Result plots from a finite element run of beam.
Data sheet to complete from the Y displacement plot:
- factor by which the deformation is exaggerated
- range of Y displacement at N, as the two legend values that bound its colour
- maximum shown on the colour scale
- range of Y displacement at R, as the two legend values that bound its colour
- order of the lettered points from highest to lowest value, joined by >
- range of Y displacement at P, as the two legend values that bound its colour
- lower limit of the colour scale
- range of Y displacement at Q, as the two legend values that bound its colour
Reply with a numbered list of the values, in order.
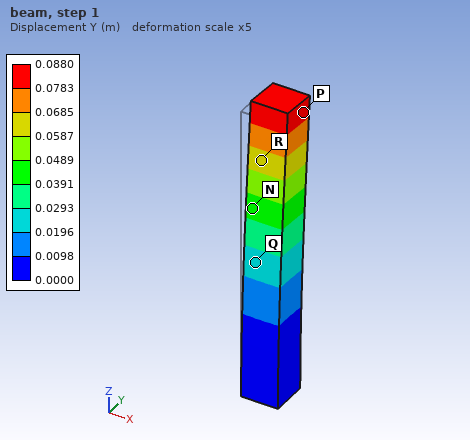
1. 5
2. 0.0391 to 0.0489 m
3. 0.0880 m
4. 0.0587 to 0.0685 m
5. P > R > N > Q
6. 0.0783 to 0.0880 m
7. 0.0000 m
8. 0.0196 to 0.0293 m
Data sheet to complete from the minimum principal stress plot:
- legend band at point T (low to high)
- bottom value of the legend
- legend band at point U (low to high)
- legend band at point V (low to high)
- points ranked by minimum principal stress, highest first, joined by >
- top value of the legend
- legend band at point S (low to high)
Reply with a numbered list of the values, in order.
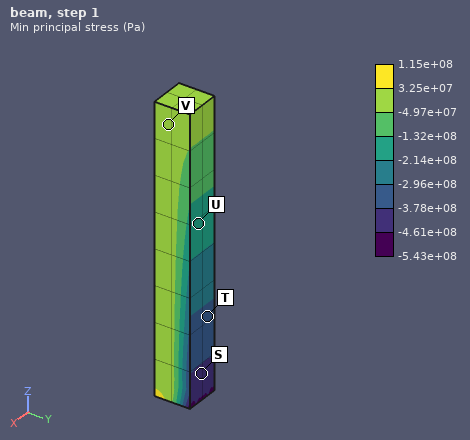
1. -3.78e+08 to -2.96e+08 Pa
2. -5.43e+08 Pa
3. -2.14e+08 to -1.32e+08 Pa
4. -4.97e+07 to 3.25e+07 Pa
5. V > U > T > S
6. 1.15e+08 Pa
7. -4.61e+08 to -3.78e+08 Pa
